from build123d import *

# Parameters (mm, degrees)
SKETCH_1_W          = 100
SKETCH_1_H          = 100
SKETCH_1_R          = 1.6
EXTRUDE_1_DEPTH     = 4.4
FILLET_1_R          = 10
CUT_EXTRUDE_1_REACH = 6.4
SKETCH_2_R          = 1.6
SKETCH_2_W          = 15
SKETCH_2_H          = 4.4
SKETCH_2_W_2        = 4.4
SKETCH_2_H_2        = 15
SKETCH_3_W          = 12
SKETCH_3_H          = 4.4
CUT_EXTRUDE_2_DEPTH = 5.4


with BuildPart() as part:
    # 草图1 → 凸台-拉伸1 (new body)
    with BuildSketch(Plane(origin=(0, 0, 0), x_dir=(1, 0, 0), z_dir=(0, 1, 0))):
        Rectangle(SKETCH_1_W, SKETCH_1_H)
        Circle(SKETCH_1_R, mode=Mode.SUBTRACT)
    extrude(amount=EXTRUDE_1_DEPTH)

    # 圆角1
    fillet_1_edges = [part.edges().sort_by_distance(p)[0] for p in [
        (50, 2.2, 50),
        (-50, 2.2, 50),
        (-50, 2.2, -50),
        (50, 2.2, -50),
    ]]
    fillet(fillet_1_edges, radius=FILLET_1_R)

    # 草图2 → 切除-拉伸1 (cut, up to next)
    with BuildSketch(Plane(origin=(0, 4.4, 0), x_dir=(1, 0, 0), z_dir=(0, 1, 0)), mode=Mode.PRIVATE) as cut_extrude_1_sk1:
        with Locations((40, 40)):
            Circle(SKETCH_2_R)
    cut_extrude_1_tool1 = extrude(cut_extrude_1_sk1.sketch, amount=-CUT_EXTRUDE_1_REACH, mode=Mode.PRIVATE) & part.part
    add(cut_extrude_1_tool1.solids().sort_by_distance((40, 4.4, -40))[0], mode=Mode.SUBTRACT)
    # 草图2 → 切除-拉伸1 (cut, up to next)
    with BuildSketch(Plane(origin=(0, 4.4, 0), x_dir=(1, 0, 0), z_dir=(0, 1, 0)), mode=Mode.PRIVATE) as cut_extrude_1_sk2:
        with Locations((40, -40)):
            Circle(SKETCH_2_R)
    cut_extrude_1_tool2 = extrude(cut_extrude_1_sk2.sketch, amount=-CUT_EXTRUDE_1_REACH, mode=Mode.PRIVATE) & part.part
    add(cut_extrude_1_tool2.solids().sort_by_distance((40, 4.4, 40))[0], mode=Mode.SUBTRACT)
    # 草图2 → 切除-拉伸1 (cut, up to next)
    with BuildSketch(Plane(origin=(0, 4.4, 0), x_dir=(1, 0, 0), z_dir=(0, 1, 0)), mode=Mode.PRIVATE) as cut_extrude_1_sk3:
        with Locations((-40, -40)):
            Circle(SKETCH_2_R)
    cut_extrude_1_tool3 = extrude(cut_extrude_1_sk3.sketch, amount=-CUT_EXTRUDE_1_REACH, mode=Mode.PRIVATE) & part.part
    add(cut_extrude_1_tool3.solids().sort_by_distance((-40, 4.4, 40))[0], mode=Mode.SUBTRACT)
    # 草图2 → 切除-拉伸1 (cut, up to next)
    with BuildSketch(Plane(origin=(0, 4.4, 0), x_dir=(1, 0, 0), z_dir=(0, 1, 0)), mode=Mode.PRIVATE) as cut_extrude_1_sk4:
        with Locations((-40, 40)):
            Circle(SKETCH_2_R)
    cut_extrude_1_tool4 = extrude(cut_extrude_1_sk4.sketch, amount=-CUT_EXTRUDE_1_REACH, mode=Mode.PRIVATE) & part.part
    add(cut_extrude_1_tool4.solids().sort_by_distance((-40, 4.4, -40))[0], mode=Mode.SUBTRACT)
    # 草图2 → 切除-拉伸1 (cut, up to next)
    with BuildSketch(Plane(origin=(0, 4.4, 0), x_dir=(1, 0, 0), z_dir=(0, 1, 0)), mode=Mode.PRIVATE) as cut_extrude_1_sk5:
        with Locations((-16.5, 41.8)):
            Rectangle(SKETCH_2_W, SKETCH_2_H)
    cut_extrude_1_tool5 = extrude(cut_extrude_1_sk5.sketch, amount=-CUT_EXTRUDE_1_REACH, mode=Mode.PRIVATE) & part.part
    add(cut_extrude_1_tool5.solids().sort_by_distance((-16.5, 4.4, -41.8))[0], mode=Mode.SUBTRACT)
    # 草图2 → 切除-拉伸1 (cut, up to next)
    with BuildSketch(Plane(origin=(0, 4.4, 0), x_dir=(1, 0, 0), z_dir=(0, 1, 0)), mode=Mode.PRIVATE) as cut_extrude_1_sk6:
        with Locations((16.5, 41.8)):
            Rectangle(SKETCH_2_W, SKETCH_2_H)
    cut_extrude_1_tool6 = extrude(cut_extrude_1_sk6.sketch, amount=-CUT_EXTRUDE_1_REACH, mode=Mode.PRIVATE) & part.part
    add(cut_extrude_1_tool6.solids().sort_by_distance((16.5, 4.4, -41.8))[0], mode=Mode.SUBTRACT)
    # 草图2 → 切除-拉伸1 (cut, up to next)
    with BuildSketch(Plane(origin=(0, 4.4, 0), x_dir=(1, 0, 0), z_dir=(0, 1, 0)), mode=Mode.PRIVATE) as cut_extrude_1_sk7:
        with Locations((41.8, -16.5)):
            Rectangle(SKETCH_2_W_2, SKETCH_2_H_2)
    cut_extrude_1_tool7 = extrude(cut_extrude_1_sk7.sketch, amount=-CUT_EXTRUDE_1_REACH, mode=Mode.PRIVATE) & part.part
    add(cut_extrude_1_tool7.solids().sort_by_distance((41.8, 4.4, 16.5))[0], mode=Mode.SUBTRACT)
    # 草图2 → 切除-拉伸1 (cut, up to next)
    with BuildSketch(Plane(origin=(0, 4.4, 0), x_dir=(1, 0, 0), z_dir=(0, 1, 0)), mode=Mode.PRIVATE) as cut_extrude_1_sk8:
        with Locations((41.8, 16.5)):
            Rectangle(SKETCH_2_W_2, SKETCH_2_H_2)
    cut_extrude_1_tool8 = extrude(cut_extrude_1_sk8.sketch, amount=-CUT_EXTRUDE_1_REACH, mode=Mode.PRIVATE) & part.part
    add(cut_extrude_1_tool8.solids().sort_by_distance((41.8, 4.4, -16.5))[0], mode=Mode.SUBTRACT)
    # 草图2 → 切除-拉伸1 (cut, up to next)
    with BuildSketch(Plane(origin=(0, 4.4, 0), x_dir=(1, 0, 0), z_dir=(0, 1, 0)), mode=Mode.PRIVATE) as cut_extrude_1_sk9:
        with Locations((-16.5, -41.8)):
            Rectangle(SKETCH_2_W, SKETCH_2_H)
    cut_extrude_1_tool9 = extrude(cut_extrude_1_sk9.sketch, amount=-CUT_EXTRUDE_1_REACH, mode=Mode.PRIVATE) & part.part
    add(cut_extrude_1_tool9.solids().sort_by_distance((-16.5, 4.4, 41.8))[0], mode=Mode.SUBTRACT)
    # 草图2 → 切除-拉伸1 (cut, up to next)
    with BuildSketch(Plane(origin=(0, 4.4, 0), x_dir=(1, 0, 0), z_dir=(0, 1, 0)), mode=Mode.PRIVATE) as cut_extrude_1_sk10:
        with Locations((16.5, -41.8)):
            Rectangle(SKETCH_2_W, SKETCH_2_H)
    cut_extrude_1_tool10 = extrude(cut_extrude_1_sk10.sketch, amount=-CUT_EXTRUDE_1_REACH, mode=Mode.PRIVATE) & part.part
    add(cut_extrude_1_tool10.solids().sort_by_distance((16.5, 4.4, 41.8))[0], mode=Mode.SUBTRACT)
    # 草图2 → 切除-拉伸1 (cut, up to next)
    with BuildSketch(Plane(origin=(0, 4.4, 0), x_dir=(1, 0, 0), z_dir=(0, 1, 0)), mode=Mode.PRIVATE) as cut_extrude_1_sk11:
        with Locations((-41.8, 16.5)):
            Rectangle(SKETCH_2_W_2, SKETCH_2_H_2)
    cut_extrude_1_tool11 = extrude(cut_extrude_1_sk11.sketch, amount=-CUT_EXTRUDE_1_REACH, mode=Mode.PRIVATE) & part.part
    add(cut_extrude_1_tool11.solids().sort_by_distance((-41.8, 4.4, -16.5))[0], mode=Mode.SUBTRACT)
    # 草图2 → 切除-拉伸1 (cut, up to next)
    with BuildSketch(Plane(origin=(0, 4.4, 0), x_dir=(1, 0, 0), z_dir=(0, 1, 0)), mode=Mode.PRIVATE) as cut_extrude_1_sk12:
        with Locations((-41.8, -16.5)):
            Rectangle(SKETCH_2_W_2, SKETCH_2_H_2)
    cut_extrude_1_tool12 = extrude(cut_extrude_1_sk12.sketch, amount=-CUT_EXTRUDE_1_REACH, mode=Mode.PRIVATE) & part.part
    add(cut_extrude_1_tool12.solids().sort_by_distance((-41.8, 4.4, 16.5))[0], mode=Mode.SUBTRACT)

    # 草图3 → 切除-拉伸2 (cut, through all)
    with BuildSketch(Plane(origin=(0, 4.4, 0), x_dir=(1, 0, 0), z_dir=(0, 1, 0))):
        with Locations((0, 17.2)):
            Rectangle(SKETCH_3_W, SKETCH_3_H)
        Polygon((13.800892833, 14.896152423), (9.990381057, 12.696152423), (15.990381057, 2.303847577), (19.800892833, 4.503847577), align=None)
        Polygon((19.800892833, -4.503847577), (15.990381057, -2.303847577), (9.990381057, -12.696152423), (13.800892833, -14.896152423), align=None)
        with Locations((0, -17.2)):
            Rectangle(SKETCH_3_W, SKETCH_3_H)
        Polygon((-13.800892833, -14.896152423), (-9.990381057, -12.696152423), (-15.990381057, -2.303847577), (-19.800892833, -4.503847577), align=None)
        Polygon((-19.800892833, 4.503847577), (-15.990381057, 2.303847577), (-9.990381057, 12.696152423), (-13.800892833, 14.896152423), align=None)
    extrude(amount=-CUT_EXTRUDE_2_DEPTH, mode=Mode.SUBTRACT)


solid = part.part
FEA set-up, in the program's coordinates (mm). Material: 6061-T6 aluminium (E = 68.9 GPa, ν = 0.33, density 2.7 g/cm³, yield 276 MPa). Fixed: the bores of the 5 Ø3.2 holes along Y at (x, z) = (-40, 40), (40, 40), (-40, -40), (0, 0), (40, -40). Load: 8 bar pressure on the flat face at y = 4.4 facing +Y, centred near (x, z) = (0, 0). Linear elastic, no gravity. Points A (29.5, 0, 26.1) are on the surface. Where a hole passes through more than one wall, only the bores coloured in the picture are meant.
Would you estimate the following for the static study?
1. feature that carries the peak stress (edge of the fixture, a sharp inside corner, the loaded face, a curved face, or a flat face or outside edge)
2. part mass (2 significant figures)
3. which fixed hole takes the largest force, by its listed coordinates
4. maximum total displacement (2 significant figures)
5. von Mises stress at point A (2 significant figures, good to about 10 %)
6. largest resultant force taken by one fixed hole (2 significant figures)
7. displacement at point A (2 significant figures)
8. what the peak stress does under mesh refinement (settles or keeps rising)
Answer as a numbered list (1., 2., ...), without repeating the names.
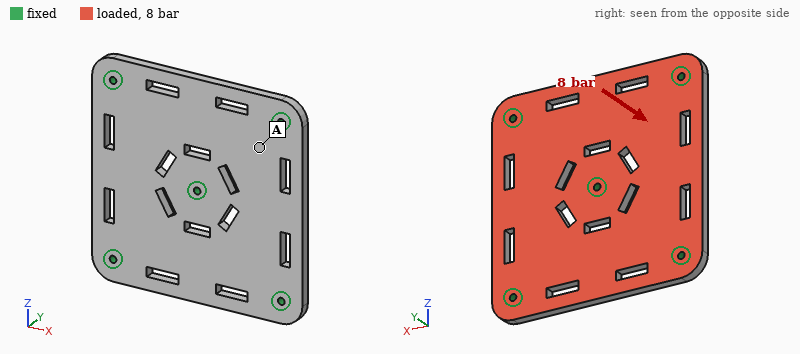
1. edge of the fixture
2. 110 g
3. (0, 0)
4. 0.14 mm
5. 49 MPa
6. 2.4 kN
7. 0.065 mm
8. keeps rising
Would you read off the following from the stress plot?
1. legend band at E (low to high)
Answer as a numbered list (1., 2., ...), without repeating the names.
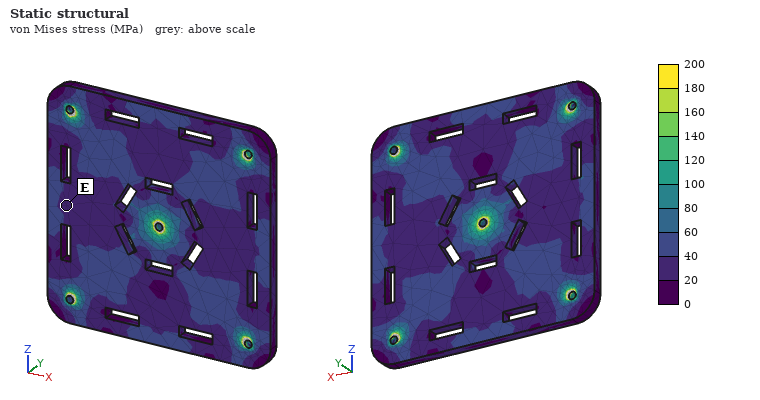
1. 20 to 40 MPa
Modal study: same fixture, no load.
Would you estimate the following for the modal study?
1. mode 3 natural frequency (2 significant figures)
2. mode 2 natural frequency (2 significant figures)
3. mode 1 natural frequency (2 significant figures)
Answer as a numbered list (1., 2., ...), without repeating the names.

1. 3900 Hz
2. 3900 Hz
3. 3800 Hz
